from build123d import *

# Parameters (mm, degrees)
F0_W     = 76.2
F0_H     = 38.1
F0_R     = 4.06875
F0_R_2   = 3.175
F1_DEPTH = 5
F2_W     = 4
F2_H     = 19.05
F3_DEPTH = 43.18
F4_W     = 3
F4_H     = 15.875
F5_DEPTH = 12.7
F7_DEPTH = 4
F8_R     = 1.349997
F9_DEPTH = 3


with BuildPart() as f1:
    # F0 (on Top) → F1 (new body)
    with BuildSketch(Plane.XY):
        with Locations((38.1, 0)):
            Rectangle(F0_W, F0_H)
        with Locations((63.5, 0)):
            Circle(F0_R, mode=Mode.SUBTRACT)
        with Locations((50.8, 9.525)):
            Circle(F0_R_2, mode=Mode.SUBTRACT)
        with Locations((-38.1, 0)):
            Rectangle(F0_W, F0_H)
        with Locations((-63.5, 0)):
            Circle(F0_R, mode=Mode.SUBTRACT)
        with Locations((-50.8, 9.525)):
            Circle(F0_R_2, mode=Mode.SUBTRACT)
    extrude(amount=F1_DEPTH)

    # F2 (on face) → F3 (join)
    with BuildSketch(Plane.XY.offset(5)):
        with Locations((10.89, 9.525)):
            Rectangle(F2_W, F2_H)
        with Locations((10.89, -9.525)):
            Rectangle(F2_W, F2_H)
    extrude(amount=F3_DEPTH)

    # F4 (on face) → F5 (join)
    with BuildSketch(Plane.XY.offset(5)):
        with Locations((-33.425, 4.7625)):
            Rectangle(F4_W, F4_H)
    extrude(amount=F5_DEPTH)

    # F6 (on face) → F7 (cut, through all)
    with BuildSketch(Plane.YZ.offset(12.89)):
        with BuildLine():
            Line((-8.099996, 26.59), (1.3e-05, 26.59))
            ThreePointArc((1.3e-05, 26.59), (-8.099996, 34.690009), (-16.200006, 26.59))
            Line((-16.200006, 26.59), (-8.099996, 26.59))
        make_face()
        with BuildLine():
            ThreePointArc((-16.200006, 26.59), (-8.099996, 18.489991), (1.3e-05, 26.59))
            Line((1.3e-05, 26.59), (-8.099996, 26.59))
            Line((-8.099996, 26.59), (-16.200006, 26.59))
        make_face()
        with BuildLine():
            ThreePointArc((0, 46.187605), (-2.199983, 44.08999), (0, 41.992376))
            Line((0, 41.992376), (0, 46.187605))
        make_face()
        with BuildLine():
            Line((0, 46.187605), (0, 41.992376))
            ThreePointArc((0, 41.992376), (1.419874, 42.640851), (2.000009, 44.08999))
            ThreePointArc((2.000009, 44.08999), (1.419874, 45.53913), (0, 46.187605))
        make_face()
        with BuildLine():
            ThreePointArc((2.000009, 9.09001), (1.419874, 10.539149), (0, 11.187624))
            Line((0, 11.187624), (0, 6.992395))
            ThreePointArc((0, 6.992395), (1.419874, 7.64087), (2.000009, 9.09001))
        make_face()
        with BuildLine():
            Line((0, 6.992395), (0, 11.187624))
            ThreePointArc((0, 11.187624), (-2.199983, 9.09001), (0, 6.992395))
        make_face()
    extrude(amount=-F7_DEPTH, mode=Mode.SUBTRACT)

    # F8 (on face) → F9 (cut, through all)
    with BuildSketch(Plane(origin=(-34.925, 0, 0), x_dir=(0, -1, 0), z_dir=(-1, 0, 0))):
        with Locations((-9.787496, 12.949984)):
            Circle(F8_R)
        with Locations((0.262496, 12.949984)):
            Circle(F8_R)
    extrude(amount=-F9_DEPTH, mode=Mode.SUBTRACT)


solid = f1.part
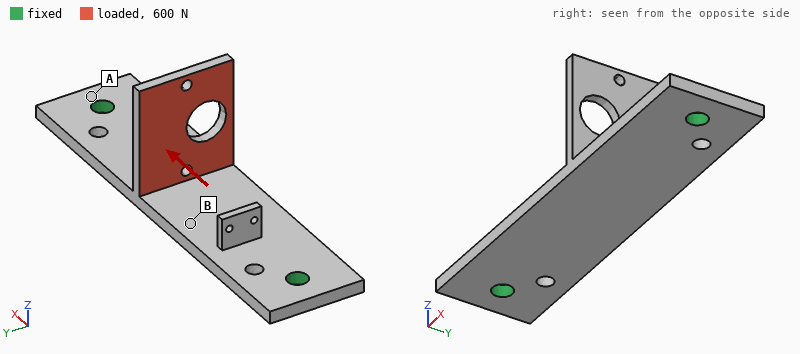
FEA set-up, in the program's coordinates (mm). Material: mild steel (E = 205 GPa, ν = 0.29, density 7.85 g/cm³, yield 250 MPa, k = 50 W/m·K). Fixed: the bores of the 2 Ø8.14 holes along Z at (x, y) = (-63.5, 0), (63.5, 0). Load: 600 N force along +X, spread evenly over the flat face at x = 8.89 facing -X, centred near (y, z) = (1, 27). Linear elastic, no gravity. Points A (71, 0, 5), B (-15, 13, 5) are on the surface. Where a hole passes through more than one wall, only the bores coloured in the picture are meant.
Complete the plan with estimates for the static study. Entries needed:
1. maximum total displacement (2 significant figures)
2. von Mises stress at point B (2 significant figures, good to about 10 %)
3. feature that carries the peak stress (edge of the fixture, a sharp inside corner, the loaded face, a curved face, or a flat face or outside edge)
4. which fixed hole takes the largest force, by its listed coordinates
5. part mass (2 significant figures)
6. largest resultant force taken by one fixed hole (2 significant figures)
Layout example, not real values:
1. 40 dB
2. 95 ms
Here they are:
1. 0.26 mm
2. 24 MPa
3. a curved face
4. (63.5, 0)
5. 270 g
6. 380 N
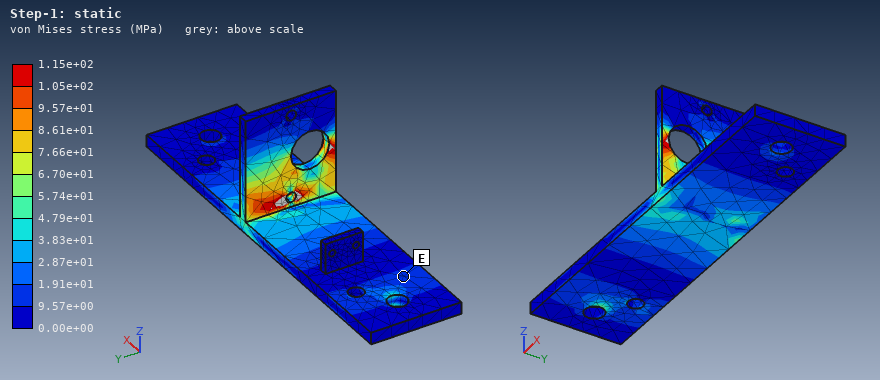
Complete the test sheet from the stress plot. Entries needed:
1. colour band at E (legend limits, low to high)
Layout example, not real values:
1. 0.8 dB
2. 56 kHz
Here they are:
1. 9.57e+00 to 1.91e+01 MPa
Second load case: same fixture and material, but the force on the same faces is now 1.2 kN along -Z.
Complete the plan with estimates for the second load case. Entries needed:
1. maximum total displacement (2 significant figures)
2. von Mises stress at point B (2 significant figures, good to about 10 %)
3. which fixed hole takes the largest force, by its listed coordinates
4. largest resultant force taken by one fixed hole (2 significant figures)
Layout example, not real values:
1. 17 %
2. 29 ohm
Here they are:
1. 0.19 mm
2. 47 MPa
3. (63.5, 0)
4. 730 N
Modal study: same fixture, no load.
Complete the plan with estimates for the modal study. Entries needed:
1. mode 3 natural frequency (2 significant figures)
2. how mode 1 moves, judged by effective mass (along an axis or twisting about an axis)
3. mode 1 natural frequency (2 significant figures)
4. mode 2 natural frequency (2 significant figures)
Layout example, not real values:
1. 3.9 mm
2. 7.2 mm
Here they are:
1. 1500 Hz
2. along Z
3. 1300 Hz
4. 1500 Hz
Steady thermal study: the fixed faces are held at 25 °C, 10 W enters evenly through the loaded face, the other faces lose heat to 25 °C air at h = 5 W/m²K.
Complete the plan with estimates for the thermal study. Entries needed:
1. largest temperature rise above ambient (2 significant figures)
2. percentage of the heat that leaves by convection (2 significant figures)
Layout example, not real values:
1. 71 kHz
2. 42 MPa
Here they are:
1. 68 K
2. 15 %
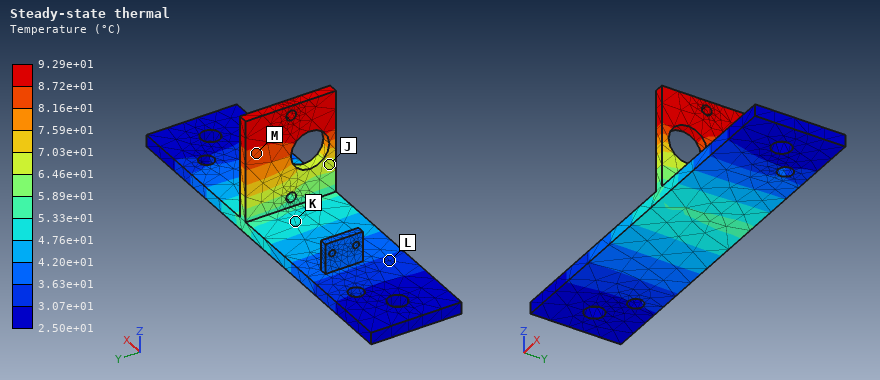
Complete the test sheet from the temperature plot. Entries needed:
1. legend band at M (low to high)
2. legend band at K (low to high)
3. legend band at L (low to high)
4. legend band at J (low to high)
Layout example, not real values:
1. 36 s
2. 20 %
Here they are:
1. 8.16e+01 to 8.72e+01 °C
2. 4.76e+01 to 5.33e+01 °C
3. 3.07e+01 to 3.63e+01 °C
4. 6.46e+01 to 7.03e+01 °C
